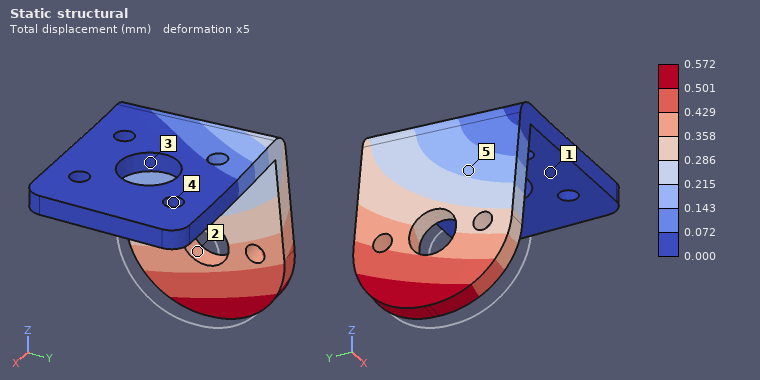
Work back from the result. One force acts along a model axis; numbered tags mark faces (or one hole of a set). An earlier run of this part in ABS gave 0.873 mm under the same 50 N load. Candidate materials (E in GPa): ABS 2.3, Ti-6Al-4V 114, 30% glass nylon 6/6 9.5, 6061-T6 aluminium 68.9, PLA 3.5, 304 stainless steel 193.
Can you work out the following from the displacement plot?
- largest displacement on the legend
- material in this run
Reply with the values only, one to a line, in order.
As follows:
0.572 mm
PLA
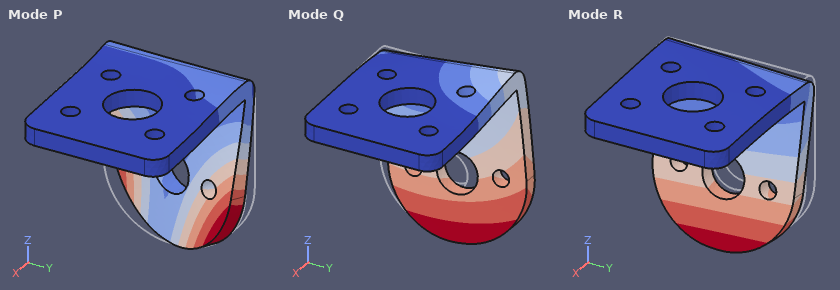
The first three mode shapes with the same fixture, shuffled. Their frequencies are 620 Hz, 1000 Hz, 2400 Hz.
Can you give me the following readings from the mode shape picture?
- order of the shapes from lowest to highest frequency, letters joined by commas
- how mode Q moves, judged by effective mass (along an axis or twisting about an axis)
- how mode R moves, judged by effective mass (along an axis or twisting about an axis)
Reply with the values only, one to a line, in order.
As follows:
R, Q, P
along Y
along X
